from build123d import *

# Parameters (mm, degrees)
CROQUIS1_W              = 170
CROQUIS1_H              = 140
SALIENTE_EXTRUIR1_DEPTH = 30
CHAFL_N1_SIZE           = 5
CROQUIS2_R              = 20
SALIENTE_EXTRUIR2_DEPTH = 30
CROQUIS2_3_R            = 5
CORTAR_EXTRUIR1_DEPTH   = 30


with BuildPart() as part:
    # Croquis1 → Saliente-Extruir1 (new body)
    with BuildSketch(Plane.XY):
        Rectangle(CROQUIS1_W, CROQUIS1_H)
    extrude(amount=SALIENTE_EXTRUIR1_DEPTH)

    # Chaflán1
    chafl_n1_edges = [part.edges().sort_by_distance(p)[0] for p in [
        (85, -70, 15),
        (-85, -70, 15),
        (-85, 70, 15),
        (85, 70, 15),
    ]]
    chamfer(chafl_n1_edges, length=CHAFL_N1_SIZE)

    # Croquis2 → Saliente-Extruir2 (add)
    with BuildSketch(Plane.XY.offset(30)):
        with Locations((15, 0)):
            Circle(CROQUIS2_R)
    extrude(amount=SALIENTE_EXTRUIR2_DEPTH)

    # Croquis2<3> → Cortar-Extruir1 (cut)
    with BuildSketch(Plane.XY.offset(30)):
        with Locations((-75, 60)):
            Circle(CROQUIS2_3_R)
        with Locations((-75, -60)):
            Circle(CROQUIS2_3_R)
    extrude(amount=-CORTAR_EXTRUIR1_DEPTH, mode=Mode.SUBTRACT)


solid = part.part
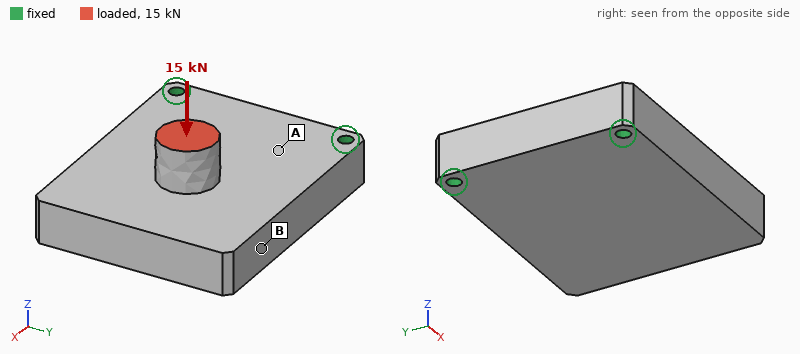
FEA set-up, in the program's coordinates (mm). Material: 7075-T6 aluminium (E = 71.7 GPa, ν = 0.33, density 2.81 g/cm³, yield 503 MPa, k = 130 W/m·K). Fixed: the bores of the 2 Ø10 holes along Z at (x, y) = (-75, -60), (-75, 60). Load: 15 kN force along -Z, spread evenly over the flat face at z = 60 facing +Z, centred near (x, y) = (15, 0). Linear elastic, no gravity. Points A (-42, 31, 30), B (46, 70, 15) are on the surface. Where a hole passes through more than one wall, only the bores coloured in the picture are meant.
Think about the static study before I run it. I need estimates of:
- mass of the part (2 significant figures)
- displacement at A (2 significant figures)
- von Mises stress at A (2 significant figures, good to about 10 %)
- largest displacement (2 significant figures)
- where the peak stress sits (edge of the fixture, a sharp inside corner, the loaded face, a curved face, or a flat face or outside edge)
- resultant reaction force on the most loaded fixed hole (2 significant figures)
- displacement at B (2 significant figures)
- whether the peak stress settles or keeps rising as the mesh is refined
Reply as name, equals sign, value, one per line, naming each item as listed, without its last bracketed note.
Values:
mass of the part = 2.1 kg
displacement at A = 0.10 mm
von Mises stress at A = 37 MPa
largest displacement = 0.65 mm
where the peak stress sits = edge of the fixture
resultant reaction force on the most loaded fixed hole = 7.5 kN
displacement at B = 0.45 mm
whether the peak stress settles or keeps rising as the mesh is refined = keeps rising
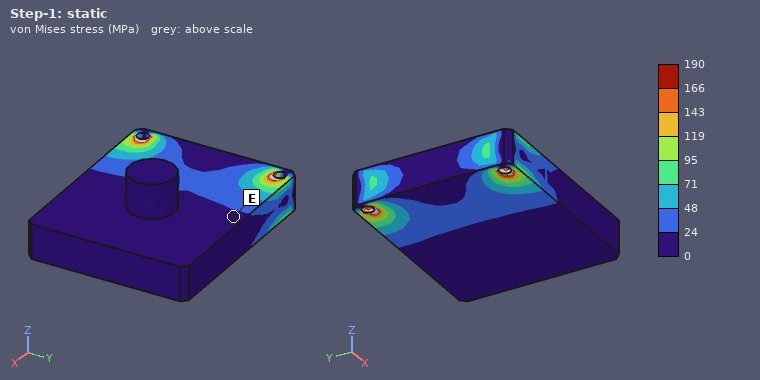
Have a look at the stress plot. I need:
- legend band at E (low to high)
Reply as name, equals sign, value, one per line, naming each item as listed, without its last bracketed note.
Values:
legend band at E = 0 to 24 MPa
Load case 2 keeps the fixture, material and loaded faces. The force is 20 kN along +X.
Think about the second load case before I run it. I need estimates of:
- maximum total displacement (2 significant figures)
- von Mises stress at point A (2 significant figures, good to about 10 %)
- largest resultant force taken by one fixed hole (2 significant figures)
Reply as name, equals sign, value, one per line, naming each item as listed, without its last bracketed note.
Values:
maximum total displacement = 0.59 mm
von Mises stress at point A = 42 MPa
largest resultant force taken by one fixed hole = 11 kN
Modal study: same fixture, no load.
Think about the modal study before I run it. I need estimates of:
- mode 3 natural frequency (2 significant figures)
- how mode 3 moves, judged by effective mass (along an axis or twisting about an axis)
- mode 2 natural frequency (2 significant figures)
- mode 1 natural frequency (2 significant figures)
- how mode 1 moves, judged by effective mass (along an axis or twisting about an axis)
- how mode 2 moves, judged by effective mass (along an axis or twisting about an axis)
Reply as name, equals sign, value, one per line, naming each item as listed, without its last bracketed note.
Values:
mode 3 natural frequency = 2900 Hz
how mode 3 moves, judged by effective mass = along Y
mode 2 natural frequency = 2300 Hz
mode 1 natural frequency = 710 Hz
how mode 1 moves, judged by effective mass = along Z
how mode 2 moves, judged by effective mass = twisting about X
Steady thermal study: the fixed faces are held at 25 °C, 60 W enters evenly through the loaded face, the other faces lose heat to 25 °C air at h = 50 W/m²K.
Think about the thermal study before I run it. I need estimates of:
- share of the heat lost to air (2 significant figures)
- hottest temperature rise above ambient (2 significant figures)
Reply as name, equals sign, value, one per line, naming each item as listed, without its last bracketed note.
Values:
share of the heat lost to air = 36 %
hottest temperature rise above ambient = 22 K
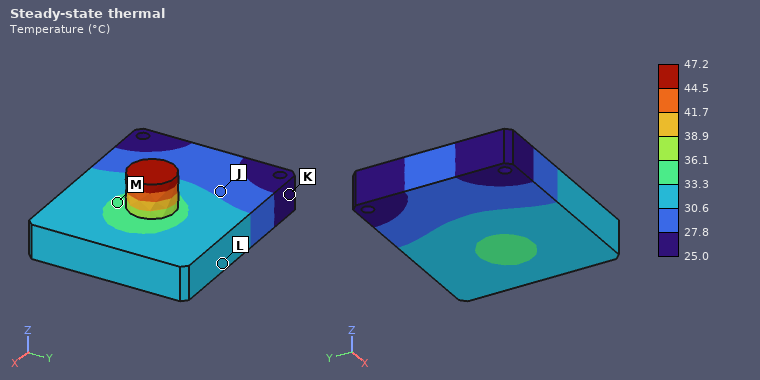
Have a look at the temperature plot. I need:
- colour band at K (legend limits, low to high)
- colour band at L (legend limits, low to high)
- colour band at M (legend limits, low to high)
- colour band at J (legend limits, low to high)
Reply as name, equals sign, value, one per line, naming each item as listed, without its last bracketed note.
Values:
colour band at K = 25.0 to 27.8 °C
colour band at L = 30.6 to 33.3 °C
colour band at M = 33.3 to 36.1 °C
colour band at J = 27.8 to 30.6 °C
